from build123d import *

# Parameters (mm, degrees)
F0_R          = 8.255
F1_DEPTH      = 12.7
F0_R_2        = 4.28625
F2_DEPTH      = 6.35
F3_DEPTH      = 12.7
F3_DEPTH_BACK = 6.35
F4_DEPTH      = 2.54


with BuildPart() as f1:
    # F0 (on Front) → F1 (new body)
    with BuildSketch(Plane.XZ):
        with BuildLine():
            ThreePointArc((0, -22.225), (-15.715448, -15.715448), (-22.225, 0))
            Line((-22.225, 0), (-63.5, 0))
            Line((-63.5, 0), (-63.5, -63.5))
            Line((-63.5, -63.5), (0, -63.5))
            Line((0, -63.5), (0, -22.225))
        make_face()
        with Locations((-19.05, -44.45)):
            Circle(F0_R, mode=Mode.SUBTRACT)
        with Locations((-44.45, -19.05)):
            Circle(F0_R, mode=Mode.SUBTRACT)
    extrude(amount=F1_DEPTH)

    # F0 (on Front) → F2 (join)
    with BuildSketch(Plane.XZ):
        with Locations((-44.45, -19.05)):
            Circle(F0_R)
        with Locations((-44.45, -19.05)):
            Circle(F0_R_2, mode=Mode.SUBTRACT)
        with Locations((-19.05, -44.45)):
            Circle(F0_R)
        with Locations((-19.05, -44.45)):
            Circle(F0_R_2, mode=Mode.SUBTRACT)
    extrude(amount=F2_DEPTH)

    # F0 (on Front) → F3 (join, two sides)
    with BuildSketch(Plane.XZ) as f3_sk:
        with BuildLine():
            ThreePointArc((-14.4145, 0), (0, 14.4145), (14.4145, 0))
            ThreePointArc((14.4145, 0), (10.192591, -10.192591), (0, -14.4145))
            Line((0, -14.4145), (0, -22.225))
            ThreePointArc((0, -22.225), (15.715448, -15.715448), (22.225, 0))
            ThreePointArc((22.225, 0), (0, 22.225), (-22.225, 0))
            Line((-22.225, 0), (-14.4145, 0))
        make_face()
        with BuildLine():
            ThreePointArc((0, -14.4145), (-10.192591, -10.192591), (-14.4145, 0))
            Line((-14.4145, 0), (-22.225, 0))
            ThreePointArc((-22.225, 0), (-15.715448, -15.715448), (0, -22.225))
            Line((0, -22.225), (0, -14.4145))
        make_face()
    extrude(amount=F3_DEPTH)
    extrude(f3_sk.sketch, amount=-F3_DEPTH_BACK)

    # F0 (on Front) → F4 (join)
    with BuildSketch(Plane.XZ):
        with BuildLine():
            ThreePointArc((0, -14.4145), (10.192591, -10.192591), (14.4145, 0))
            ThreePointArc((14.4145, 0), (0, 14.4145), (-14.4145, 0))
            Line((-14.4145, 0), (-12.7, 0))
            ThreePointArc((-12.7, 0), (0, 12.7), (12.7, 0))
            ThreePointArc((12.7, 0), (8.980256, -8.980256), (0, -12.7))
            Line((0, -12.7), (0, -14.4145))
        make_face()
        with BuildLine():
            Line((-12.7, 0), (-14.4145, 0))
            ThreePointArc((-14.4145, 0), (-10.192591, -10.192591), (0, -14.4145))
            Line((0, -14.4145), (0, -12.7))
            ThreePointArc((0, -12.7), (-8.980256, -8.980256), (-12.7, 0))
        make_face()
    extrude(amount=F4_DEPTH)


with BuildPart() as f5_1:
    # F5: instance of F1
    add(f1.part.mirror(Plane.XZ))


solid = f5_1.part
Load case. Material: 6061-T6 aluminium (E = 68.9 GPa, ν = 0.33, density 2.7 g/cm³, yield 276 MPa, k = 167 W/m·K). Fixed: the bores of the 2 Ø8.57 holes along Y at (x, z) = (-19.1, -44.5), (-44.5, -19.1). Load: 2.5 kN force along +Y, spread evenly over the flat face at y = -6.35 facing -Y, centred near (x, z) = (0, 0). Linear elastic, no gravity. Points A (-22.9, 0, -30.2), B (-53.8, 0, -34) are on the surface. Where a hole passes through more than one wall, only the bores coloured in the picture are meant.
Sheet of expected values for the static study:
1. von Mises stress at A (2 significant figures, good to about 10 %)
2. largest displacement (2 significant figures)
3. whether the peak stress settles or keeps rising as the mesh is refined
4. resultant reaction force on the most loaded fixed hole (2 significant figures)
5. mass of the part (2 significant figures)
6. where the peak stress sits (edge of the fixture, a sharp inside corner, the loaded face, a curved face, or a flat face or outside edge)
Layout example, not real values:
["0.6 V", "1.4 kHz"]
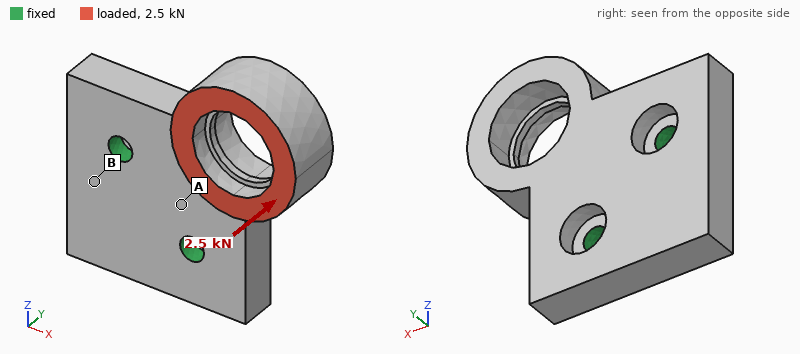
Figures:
["60 MPa", "0.43 mm", "keeps rising", "1.5 kN", "160 g", "edge of the fixture"]
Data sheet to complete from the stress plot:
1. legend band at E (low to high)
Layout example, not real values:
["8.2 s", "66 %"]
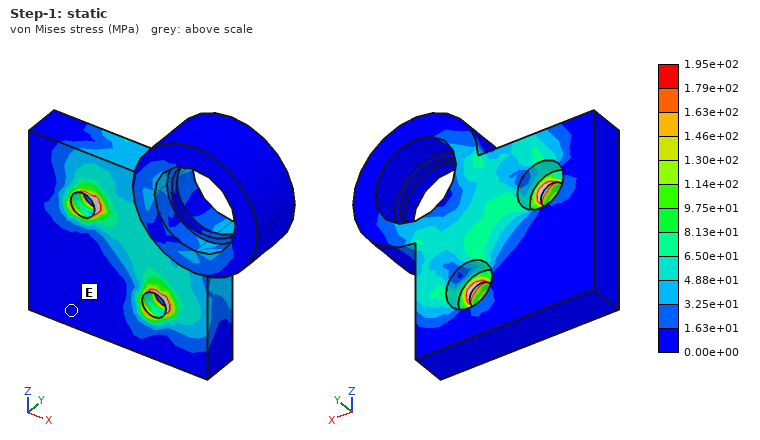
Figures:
["0.00e+00 to 1.63e+01 MPa"]
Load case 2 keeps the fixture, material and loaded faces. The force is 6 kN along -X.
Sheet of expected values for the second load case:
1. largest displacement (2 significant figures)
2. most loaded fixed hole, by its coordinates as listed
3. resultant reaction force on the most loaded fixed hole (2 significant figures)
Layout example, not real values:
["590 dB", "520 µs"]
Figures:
["0.32 mm", "(-44.5, -19.1)", "7.4 kN"]
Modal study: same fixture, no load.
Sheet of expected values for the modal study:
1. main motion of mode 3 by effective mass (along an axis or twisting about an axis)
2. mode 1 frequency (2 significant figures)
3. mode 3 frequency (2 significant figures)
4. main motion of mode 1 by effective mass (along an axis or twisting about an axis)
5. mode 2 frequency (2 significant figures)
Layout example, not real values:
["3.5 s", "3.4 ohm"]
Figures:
["along Y", "2100 Hz", "5900 Hz", "along Y", "4800 Hz"]
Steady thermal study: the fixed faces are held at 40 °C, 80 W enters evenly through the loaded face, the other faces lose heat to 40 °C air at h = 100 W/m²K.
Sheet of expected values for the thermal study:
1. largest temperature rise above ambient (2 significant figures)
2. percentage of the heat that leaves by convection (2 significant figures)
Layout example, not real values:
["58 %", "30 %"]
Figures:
["46 K", "27 %"]
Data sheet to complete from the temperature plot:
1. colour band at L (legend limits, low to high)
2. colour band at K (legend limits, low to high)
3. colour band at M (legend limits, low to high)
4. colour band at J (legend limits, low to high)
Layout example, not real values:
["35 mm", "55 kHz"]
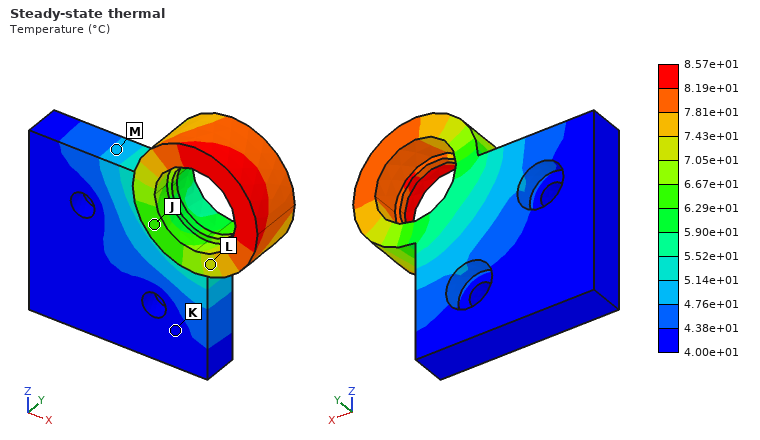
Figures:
["7.05e+01 to 7.43e+01 °C", "4.00e+01 to 4.38e+01 °C", "4.76e+01 to 5.14e+01 °C", "6.29e+01 to 6.67e+01 °C"]
